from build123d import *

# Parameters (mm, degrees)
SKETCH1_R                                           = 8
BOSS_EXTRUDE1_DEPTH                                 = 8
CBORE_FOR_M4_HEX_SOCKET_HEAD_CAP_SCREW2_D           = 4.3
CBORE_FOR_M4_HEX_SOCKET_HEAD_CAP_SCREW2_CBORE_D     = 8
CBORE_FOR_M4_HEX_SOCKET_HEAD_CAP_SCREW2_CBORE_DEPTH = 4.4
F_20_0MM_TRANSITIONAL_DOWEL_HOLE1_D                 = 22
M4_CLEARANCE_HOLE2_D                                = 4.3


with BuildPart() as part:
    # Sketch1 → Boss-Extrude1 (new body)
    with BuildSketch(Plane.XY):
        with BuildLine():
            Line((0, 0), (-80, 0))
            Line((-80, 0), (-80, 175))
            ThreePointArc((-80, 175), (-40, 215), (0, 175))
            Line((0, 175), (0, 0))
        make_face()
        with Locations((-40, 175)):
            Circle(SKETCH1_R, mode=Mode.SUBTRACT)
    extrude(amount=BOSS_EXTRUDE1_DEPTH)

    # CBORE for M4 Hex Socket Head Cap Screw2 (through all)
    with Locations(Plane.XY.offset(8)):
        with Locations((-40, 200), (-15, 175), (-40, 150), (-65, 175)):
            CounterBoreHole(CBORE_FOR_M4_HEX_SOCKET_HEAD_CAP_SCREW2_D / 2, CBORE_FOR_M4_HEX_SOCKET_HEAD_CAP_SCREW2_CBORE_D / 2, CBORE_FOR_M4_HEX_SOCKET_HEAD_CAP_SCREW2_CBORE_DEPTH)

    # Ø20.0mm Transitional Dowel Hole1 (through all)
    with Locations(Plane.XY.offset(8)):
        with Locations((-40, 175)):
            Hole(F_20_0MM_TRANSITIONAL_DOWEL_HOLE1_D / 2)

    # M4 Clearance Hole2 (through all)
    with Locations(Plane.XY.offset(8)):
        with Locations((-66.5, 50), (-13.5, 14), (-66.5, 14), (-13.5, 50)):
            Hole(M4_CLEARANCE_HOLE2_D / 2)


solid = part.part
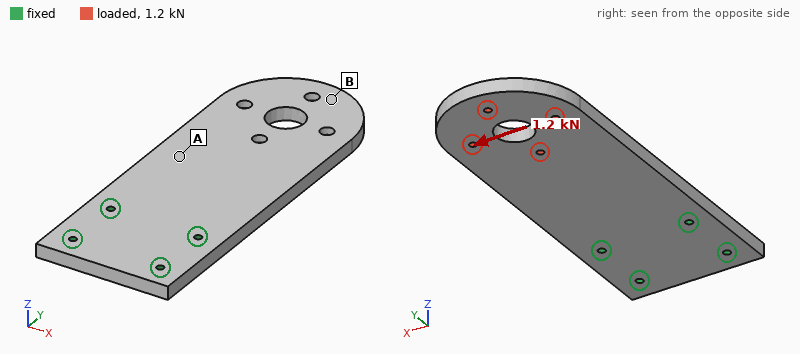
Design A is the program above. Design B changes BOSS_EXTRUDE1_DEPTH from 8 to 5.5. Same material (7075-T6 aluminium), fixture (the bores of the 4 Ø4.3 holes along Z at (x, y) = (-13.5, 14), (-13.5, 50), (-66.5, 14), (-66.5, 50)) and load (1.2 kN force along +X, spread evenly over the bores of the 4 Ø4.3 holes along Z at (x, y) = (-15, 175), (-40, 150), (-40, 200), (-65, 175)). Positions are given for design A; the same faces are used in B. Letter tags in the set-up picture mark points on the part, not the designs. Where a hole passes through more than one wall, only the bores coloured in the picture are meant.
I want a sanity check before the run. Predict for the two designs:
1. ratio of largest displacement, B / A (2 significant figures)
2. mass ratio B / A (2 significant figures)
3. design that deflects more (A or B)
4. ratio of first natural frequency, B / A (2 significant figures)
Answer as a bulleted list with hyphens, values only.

- 1.4
- 0.69
- B
- 0.69
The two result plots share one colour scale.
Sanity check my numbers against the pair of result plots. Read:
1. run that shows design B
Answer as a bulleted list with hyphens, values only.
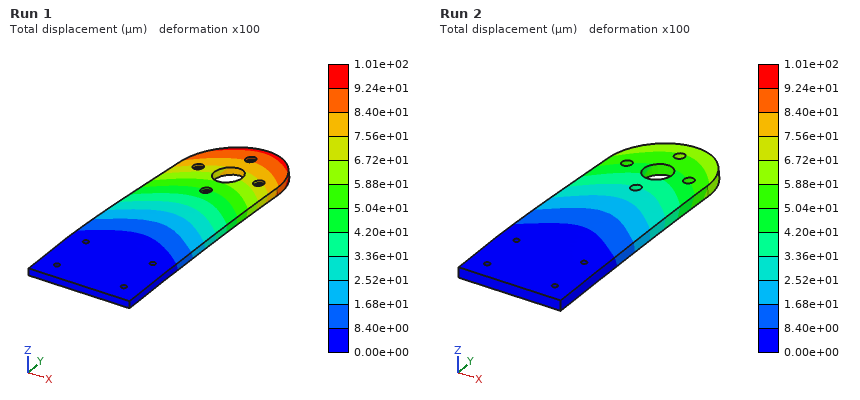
- Run 1
